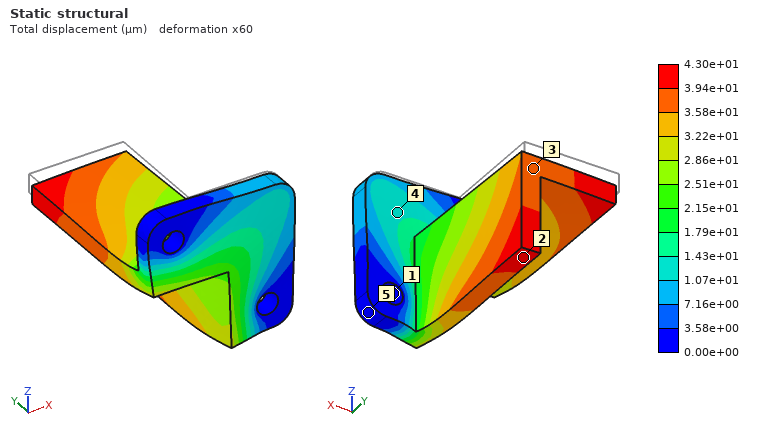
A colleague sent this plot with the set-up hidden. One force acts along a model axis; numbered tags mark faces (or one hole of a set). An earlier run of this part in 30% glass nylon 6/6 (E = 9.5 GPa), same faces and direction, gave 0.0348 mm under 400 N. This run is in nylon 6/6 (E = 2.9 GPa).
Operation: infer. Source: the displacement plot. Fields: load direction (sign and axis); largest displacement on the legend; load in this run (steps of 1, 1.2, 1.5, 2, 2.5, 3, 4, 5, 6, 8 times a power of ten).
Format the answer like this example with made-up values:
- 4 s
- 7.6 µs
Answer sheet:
- -Y
- 4.30e+01 µm
- 150 N
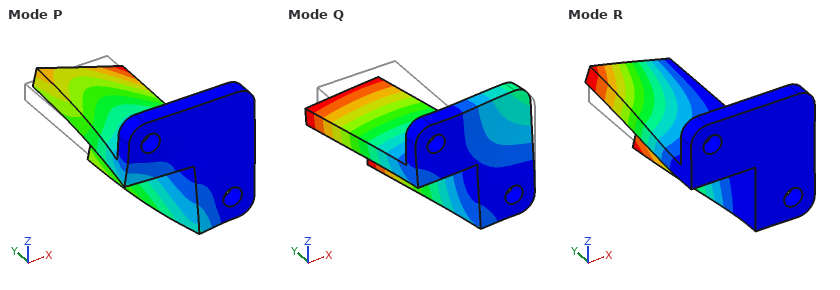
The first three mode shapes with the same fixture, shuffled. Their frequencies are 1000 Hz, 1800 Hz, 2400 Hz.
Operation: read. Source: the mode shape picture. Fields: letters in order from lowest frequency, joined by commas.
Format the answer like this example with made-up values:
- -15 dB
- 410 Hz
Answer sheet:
- Q, R, P
